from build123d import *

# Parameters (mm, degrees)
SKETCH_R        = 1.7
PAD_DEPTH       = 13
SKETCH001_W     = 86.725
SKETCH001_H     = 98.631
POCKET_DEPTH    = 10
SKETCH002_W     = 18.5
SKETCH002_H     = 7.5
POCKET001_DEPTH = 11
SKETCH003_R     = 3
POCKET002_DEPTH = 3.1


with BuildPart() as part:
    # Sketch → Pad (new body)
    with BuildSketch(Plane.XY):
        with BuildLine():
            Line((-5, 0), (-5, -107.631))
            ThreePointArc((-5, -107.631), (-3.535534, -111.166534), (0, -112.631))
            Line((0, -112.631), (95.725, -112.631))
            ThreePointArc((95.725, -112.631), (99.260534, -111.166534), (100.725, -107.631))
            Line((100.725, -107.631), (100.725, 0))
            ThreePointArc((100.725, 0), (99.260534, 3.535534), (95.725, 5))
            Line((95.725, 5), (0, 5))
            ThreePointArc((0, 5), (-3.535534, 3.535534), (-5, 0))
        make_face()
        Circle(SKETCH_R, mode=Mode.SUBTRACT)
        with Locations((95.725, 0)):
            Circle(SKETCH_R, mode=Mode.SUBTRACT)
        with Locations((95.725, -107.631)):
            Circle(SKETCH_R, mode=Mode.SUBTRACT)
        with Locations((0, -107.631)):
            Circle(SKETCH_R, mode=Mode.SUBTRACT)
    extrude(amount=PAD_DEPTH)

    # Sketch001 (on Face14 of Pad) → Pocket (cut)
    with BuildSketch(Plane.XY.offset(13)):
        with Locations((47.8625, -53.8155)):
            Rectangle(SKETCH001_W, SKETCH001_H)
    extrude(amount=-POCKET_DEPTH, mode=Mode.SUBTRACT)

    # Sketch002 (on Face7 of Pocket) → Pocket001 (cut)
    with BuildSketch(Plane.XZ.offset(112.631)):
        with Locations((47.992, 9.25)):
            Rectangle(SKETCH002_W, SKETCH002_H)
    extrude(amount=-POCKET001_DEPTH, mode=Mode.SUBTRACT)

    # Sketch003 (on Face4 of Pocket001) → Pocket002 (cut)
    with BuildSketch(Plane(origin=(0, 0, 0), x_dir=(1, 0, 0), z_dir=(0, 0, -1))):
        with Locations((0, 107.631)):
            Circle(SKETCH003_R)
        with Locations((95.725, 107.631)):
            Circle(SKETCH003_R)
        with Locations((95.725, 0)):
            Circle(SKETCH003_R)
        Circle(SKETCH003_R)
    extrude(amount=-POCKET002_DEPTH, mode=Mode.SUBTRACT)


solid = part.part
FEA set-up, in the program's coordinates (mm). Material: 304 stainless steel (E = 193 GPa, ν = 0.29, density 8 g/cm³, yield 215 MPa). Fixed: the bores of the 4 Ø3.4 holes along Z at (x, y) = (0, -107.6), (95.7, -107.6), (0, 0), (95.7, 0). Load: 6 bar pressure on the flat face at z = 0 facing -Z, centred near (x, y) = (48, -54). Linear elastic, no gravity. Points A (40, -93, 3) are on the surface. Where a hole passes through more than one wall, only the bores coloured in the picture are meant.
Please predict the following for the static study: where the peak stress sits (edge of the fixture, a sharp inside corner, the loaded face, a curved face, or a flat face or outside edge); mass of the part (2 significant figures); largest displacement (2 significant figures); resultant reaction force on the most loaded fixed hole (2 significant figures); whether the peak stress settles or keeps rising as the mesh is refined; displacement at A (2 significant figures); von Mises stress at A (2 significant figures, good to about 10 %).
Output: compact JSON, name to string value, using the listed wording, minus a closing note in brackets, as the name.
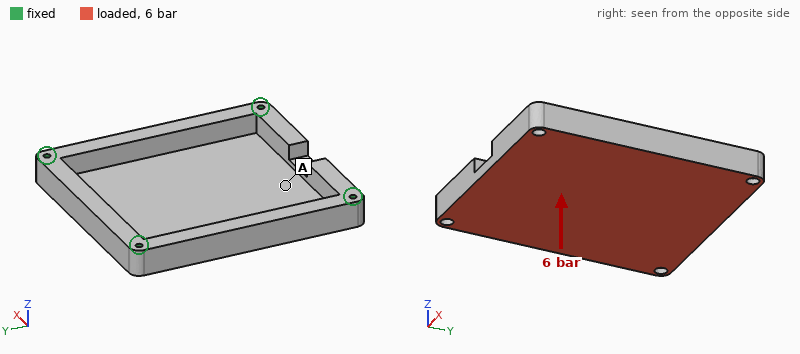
{"where the peak stress sits": "edge of the fixture", "mass of the part": "590 g", "largest displacement": "0.20 mm", "resultant reaction force on the most loaded fixed hole": "3.4 kN", "whether the peak stress settles or keeps rising as the mesh is refined": "keeps rising", "displacement at A": "0.070 mm", "von Mises stress at A": "38 MPa"}
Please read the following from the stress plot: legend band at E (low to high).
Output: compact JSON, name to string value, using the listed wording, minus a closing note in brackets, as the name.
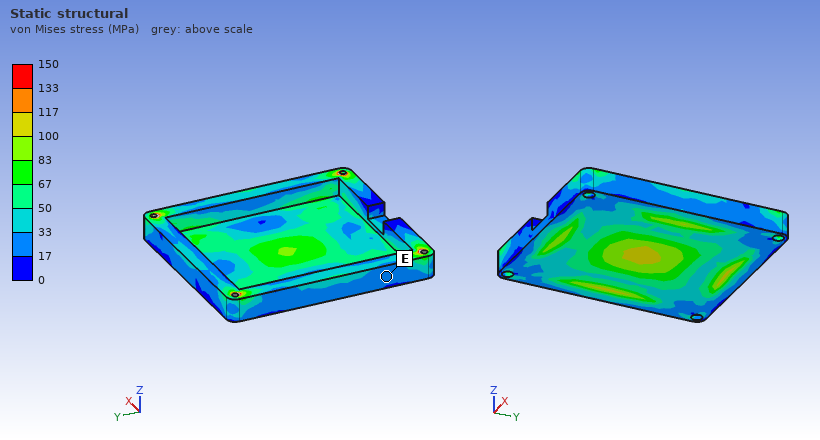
{"legend band at E": "17 to 33 MPa"}
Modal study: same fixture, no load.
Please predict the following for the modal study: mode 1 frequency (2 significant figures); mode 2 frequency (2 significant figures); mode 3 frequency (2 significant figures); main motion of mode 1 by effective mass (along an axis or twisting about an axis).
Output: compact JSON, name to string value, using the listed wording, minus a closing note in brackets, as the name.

{"mode 1 frequency": "2300 Hz", "mode 2 frequency": "4000 Hz", "mode 3 frequency": "4100 Hz", "main motion of mode 1 by effective mass": "along Z"}
